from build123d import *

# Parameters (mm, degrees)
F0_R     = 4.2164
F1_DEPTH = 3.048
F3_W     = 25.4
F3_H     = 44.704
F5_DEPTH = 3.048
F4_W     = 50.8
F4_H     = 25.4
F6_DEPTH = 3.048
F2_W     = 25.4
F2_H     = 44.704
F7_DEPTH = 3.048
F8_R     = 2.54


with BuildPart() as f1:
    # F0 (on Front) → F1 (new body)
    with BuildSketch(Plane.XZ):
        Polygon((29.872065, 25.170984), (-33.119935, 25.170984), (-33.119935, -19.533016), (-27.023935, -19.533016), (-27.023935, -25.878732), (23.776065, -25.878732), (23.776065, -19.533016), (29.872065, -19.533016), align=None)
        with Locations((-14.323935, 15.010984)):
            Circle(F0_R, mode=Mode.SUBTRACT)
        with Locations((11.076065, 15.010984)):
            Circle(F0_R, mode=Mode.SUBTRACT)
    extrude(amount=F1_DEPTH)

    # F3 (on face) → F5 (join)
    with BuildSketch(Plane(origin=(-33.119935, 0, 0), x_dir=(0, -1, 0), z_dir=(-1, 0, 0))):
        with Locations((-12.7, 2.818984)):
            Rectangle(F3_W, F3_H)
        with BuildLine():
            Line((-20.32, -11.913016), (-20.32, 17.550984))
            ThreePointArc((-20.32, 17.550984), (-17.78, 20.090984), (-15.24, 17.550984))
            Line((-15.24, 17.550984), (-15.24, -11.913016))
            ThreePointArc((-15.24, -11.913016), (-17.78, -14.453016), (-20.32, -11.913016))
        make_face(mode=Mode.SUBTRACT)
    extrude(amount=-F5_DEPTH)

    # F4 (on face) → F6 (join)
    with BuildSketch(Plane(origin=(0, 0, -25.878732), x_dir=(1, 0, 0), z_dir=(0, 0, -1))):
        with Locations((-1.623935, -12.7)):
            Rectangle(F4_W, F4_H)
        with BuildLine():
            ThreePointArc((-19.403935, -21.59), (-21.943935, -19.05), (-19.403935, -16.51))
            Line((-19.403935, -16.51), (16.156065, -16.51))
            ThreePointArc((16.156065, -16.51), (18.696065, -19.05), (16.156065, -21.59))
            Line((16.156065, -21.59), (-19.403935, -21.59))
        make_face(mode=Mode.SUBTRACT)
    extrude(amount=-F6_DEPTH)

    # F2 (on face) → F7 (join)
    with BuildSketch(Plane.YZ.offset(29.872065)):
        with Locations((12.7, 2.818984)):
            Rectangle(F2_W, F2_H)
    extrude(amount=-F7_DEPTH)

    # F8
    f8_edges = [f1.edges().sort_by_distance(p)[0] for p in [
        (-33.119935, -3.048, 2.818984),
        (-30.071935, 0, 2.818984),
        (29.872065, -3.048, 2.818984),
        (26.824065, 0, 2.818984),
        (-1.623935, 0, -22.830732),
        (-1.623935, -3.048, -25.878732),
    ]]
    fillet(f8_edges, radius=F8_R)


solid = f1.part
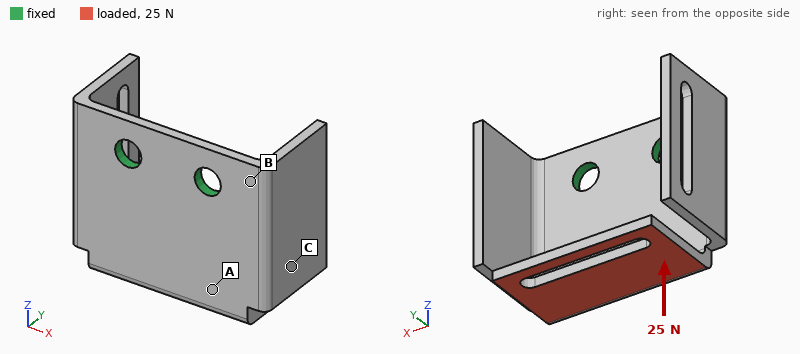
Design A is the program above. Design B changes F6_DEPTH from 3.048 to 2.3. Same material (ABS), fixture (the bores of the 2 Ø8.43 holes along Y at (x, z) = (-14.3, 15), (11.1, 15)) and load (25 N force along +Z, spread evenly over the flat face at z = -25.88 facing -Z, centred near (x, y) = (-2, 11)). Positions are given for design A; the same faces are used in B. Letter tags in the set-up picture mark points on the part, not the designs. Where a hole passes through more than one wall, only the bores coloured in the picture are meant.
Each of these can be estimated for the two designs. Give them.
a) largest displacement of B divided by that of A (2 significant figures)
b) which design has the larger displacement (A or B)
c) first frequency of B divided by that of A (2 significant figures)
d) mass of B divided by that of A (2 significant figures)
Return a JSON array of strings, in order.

["1.4", "B", "1.1", "0.96"]
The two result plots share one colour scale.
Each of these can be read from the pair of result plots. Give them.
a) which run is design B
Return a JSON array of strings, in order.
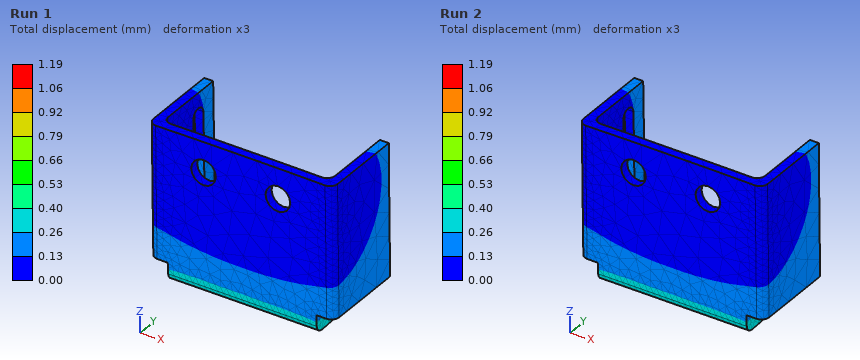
["Run 1"]
